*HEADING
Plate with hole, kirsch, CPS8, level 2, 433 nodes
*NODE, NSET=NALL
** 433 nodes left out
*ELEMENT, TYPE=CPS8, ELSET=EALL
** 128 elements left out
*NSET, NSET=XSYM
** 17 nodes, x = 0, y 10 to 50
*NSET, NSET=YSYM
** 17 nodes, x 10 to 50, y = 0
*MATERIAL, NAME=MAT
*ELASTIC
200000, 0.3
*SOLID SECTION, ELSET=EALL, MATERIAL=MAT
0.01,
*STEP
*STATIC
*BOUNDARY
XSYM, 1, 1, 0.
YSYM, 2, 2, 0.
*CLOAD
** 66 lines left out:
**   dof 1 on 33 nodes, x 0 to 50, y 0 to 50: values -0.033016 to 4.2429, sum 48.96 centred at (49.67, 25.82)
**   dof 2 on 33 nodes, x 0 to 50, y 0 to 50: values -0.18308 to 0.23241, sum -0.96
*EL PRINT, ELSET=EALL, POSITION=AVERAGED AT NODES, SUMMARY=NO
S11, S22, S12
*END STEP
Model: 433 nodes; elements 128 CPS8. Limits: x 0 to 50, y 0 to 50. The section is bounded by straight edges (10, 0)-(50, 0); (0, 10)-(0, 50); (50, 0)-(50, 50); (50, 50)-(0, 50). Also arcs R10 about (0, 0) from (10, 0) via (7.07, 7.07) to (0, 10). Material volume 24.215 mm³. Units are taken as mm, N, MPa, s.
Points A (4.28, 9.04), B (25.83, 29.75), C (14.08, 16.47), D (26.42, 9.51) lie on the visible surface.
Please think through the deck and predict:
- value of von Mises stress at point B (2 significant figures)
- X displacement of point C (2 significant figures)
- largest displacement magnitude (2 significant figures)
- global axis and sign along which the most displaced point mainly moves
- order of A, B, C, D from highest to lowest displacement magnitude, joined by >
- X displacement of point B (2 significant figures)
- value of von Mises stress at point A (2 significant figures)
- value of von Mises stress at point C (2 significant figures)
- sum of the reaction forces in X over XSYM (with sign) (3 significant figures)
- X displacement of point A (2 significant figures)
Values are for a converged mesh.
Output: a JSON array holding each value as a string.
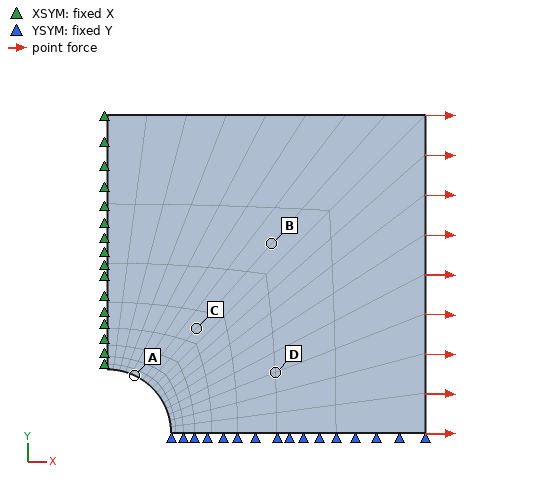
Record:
["110 MPa", "0.0090 mm", "0.029 mm", "+X", "D > B > C > A", "0.014 mm", "230 MPa", "130 MPa", "-49.0 N", "0.0064 mm"]
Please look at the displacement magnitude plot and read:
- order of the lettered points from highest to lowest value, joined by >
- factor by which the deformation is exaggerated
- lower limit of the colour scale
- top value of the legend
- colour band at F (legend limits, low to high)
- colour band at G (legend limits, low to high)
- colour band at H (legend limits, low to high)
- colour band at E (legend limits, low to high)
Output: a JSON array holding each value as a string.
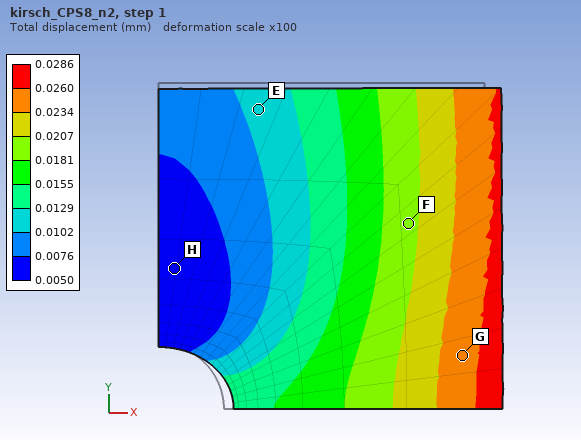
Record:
["G > F > E > H", "100", "0.0050 mm", "0.0286 mm", "0.0181 to 0.0207 mm", "0.0234 to 0.0260 mm", "0.0050 to 0.0076 mm", "0.0102 to 0.0129 mm"]
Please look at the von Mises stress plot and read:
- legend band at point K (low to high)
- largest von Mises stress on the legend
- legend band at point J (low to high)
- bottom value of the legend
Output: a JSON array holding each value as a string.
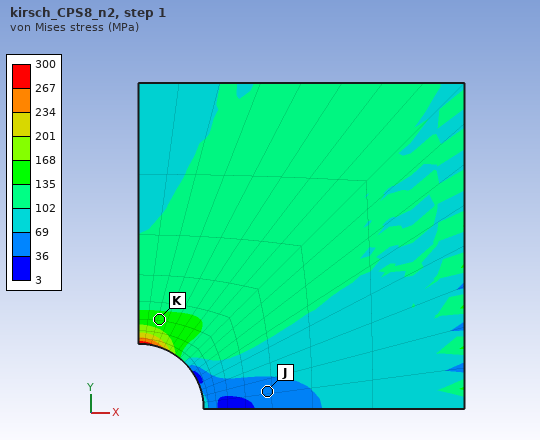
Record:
["135 to 168 MPa", "300 MPa", "36 to 69 MPa", "3 MPa"]
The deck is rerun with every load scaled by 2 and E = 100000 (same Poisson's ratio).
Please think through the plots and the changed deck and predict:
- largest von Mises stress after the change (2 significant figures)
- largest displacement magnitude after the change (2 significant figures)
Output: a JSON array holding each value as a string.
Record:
["600 MPa", "0.11 mm"]
